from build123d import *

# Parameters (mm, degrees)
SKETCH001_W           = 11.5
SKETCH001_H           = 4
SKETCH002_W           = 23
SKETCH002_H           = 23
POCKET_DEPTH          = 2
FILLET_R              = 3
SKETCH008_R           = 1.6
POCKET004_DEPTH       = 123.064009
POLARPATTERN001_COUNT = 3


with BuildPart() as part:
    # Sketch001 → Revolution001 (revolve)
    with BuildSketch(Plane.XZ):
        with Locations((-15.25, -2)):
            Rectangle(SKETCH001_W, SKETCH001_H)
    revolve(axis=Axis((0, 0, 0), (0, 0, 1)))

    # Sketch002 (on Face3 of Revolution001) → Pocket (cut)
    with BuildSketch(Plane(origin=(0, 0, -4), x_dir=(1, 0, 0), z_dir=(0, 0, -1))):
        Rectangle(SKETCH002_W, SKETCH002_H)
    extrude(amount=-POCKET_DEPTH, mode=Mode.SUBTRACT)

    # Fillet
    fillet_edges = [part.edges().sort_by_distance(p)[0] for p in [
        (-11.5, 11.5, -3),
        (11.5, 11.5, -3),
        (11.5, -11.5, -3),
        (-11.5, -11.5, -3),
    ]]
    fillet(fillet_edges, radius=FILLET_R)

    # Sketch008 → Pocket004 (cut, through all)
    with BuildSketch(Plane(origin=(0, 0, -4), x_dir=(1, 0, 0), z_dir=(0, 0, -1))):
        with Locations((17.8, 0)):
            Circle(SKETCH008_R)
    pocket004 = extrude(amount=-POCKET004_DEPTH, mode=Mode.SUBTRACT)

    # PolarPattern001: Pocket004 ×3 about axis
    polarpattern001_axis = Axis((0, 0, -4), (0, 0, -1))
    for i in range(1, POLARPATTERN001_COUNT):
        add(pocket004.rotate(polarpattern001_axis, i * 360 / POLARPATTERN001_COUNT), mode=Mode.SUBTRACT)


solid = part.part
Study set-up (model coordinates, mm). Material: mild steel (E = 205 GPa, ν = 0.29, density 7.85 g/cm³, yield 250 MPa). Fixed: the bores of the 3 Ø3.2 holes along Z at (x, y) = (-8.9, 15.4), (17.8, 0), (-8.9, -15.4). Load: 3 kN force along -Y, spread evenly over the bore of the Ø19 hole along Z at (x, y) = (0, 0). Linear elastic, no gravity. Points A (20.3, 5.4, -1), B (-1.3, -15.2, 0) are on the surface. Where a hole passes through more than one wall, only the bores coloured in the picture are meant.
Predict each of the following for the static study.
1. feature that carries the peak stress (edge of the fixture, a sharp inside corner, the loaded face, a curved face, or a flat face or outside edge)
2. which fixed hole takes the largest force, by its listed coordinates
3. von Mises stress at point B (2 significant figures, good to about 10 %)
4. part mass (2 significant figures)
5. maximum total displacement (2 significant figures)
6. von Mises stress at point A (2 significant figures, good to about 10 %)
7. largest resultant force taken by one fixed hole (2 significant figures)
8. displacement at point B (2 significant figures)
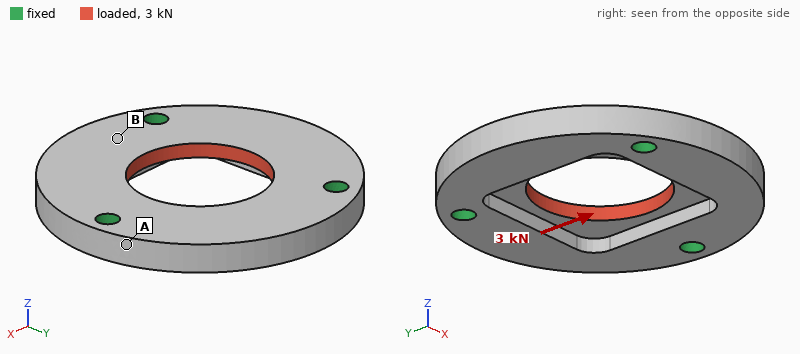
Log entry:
edge of the fixture
(17.8, 0)
30 MPa
30 g
3.8 µm
14 MPa
1.2 kN
2.0 µm
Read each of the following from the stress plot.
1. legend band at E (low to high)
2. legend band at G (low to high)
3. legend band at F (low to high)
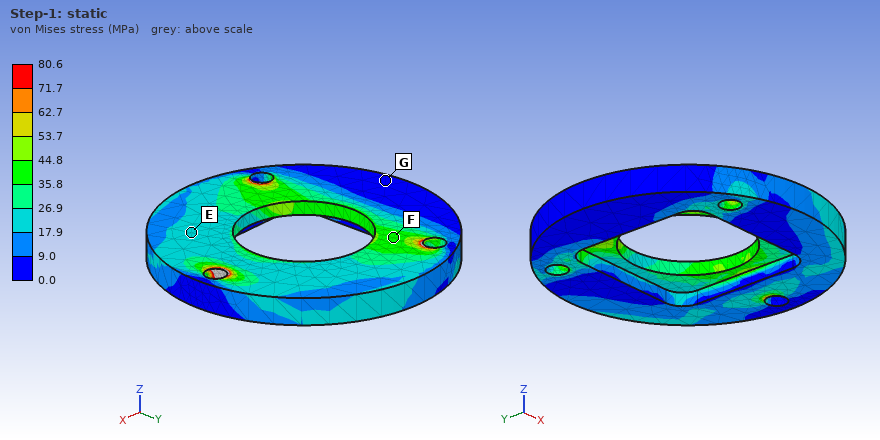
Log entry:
17.9 to 26.9 MPa
0.0 to 9.0 MPa
35.8 to 44.8 MPa
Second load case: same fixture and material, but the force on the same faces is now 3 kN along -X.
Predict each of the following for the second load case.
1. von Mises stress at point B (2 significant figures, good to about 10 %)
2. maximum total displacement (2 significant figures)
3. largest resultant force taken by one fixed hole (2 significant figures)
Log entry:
16 MPa
4.5 µm
1.1 kN
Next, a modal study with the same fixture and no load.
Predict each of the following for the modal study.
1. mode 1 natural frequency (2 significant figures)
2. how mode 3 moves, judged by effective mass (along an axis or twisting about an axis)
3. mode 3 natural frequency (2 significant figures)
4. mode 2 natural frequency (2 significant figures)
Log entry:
14 kHz
along Z
15 kHz
14 kHz
